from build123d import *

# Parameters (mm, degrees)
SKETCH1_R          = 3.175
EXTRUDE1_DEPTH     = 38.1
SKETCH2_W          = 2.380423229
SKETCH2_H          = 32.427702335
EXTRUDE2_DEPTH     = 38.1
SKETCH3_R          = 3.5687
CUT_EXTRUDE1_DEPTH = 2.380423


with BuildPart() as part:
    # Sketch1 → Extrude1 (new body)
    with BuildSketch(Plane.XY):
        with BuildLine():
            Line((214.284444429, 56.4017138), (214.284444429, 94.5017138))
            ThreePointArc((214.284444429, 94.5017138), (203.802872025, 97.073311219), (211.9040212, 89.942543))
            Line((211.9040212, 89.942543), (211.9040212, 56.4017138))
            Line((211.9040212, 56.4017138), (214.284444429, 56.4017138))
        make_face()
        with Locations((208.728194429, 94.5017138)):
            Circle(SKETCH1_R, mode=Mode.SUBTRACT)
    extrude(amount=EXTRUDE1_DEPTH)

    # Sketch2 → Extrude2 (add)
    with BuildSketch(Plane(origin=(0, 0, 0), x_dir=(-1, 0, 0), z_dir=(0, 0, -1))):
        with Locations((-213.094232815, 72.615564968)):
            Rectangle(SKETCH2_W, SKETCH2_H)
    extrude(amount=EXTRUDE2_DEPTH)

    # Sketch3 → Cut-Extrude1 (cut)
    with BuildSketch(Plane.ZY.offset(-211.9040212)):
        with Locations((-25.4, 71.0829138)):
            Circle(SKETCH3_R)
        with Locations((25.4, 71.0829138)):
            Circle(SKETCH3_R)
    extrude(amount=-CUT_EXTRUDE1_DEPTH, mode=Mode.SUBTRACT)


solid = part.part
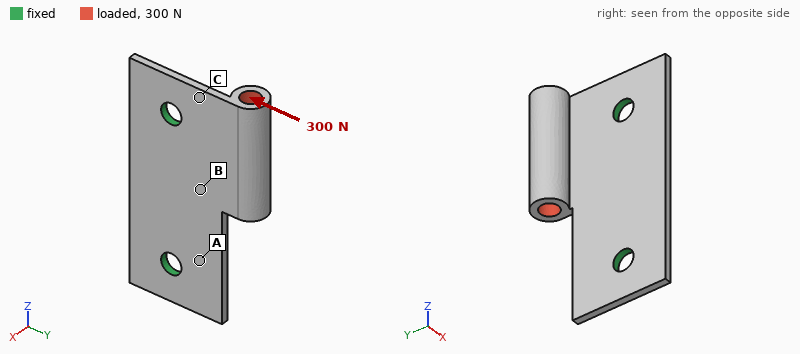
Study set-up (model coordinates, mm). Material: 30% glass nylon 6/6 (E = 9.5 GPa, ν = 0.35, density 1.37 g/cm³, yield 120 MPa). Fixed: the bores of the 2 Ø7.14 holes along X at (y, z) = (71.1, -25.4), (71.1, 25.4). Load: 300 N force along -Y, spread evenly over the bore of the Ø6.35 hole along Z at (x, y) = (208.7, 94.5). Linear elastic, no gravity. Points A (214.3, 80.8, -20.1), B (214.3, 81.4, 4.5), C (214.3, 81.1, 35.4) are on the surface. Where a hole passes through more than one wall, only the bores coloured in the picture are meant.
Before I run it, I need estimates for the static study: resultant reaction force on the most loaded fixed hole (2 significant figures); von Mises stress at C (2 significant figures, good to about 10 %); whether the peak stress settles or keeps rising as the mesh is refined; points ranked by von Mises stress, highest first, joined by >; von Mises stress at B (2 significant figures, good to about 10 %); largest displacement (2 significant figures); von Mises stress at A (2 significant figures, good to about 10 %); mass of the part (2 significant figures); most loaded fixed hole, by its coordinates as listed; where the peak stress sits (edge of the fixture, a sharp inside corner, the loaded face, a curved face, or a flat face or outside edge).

260 N
29 MPa
keeps rising
C > B > A
20 MPa
0.96 mm
7.5 MPa
12 g
(71.1, 25.4)
a sharp inside corner
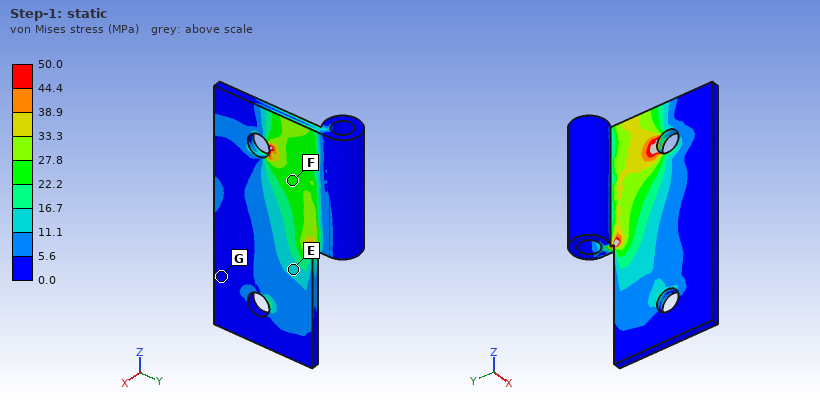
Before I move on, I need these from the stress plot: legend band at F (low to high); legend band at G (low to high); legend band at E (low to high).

22.2 to 27.8 MPa
0.0 to 5.6 MPa
11.1 to 16.7 MPa
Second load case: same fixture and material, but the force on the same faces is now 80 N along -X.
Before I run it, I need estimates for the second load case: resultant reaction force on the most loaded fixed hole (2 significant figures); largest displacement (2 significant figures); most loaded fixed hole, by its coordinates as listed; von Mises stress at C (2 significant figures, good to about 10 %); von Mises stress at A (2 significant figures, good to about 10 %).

70 N
0.87 mm
(71.1, 25.4)
26 MPa
10 MPa
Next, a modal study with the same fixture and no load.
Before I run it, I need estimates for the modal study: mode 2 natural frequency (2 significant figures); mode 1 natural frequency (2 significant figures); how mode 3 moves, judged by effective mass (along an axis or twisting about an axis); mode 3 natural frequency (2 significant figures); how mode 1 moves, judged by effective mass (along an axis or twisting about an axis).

1800 Hz
870 Hz
along X
2900 Hz
along X
